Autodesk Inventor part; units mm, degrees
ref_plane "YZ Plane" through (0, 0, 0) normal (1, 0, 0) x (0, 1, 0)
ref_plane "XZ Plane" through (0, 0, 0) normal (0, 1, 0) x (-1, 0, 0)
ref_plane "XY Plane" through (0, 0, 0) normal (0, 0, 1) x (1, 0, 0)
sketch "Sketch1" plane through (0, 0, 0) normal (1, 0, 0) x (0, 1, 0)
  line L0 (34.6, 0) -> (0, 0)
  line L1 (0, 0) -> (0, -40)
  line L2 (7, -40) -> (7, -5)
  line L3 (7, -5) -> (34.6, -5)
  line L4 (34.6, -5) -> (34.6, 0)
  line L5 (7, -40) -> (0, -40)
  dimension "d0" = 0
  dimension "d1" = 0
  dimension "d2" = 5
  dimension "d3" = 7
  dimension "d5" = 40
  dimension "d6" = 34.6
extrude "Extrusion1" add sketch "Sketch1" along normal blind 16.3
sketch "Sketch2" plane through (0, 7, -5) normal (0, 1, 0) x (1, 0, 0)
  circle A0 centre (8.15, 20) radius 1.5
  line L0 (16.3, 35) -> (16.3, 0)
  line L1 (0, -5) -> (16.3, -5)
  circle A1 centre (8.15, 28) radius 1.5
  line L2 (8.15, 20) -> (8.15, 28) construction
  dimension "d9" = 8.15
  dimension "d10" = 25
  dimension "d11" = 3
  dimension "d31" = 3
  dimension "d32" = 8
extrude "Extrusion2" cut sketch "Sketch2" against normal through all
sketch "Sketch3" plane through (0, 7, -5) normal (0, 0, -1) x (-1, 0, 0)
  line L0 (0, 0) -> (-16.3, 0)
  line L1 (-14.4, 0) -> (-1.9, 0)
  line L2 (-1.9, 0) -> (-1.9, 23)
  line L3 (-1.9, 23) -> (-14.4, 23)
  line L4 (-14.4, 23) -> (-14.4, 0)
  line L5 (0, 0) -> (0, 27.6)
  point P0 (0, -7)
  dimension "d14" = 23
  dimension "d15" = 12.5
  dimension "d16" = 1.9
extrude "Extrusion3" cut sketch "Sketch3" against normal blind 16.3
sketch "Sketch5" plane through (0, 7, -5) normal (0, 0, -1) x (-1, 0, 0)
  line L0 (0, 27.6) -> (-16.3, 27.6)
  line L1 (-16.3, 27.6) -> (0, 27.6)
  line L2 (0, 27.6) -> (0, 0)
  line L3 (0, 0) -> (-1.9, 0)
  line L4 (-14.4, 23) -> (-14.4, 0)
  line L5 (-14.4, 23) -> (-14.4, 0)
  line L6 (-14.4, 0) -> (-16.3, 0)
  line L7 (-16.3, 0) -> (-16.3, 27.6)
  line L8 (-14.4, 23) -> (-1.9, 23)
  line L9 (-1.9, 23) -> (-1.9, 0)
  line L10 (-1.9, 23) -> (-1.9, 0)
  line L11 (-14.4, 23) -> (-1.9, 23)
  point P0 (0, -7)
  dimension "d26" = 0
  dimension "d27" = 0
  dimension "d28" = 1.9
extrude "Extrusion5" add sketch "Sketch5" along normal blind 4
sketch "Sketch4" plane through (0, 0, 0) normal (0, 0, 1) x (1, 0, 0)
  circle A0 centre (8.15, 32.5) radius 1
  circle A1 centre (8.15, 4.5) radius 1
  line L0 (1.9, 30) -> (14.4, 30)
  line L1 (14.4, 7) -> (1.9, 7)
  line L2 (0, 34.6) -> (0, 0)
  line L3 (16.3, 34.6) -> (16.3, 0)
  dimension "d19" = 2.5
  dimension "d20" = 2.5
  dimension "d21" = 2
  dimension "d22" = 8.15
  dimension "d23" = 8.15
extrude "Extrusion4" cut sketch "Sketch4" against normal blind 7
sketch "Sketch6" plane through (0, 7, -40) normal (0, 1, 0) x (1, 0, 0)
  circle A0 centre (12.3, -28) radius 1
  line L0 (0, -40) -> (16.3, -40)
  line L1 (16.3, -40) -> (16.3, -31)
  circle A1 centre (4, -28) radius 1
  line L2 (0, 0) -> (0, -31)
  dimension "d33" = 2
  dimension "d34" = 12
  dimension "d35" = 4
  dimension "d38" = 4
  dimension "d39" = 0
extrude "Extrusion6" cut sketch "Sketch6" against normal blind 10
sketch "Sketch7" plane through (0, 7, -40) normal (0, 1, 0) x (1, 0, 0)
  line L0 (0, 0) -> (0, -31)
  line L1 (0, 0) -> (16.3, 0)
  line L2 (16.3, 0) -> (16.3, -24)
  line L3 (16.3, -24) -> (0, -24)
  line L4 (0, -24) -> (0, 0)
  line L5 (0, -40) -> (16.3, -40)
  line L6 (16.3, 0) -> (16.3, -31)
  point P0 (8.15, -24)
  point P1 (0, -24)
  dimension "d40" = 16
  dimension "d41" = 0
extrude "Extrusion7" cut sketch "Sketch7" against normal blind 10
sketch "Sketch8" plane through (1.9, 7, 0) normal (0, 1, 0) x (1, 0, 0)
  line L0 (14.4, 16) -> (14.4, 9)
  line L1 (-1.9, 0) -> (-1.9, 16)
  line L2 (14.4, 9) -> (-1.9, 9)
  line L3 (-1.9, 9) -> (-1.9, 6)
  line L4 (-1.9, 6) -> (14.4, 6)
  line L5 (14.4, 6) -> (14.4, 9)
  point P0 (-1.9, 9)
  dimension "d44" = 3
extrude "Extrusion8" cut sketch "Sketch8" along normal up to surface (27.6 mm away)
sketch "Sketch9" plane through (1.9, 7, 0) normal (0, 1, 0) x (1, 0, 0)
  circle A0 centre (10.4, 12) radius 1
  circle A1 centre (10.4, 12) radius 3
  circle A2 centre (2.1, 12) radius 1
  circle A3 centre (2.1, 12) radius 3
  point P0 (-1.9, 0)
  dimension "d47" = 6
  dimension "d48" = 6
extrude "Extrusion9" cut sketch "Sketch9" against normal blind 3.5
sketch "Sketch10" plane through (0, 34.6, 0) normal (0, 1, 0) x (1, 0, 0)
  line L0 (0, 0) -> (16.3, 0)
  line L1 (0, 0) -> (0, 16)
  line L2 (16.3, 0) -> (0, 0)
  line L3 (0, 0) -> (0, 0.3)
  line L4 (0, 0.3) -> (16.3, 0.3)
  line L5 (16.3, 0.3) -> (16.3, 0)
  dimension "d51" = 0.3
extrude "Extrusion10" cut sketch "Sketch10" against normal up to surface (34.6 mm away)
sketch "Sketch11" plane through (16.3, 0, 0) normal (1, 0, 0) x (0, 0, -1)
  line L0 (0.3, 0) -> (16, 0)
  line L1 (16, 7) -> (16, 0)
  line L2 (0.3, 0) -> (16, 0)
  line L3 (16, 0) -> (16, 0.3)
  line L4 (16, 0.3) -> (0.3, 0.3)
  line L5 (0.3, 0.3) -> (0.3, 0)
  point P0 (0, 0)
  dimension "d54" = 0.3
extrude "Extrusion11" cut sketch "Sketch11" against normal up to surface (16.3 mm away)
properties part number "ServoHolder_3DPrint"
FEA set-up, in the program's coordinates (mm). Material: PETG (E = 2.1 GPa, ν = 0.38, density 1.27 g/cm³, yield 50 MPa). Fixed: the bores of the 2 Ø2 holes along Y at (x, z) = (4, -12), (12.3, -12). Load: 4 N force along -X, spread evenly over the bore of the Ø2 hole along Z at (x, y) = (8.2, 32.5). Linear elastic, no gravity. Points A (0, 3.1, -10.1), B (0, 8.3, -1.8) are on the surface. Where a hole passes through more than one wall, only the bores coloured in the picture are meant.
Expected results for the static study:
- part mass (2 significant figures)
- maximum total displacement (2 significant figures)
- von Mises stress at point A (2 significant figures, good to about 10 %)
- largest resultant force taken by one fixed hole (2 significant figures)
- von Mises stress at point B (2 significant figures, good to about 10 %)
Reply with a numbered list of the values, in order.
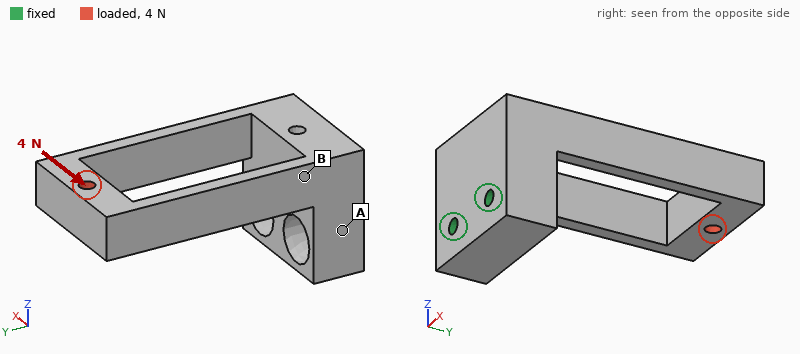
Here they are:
1. 3.0 g
2. 0.43 mm
3. 0.95 MPa
4. 12 N
5. 5.8 MPa
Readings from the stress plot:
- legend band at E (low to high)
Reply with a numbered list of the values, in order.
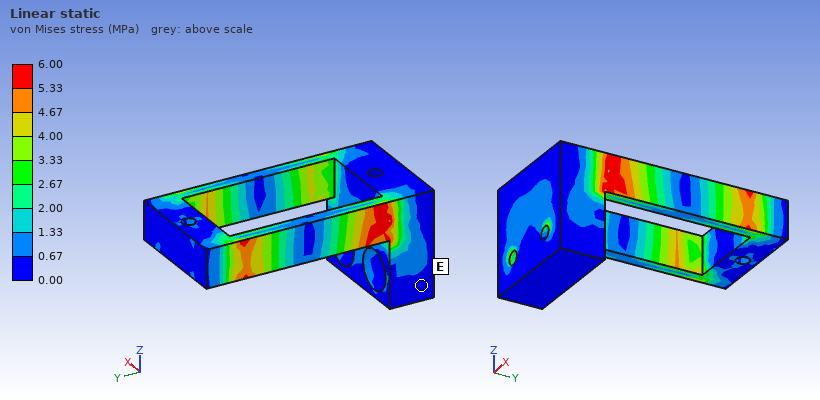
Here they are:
1. 0.00 to 0.67 MPa
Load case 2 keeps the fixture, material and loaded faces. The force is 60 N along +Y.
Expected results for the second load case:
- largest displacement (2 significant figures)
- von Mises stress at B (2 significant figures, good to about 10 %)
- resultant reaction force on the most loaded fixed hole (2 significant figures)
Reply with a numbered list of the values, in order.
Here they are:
1. 0.43 mm
2. 3.4 MPa
3. 30 N
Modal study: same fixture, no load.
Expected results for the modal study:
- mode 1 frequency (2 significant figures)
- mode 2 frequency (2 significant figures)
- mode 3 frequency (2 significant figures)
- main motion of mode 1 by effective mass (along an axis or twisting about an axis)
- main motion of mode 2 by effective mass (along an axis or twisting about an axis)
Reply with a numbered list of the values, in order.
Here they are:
1. 570 Hz
2. 680 Hz
3. 1800 Hz
4. along X
5. along Z
